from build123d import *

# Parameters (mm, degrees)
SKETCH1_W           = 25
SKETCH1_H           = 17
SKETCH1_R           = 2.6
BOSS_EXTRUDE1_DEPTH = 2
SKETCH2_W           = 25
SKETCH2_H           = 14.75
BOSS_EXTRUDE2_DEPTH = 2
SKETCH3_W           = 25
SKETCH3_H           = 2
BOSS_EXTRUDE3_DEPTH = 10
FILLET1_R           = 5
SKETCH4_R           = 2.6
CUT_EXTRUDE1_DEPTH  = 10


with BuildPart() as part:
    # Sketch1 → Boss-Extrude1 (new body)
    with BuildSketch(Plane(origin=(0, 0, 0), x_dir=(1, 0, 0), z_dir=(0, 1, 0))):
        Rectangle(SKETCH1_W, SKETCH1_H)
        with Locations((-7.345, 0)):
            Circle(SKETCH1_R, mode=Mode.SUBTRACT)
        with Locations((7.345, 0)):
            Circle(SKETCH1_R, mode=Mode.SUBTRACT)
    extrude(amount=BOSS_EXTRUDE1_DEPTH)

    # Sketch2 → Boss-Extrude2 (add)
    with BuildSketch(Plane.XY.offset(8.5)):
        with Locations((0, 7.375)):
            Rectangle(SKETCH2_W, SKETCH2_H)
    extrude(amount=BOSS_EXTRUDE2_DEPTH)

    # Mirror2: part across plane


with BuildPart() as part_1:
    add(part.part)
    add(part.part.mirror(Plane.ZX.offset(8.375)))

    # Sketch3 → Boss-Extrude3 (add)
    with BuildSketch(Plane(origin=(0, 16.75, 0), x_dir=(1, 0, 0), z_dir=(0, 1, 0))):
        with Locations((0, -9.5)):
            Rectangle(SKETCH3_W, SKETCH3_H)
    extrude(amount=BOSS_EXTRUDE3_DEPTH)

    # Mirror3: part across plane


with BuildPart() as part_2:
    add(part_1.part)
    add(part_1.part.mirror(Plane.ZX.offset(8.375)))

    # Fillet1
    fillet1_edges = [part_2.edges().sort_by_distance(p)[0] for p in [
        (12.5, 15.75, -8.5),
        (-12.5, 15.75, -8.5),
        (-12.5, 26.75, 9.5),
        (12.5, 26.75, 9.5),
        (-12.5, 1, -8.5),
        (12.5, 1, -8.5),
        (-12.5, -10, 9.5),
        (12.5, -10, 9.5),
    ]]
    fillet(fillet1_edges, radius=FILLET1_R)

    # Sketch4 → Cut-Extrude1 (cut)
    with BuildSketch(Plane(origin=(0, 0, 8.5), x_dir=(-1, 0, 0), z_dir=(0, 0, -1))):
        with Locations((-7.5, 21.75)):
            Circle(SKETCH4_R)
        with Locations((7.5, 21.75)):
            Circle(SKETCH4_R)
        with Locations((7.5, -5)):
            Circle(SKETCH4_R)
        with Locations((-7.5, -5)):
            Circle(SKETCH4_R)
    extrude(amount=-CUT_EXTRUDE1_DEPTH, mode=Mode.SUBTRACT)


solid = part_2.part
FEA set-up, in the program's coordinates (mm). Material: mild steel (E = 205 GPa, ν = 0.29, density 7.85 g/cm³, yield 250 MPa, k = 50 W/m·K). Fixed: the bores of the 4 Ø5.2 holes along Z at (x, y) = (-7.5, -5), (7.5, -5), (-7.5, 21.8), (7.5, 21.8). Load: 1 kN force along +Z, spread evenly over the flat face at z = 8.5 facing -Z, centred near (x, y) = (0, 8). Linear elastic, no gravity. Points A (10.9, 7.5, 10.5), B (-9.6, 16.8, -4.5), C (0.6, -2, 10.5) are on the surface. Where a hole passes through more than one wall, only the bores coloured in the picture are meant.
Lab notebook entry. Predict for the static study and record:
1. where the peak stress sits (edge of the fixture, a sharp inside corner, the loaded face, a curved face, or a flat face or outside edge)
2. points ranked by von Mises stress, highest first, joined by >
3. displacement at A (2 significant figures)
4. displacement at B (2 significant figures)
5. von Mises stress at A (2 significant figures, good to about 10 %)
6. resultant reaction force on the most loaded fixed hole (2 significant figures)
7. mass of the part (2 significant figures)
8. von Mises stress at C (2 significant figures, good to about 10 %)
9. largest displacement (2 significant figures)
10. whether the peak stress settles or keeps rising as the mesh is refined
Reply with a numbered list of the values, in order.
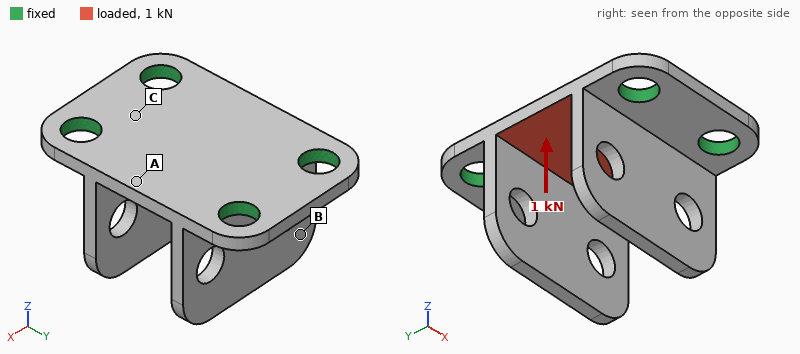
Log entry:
1. edge of the fixture
2. A > C > B
3. 16 µm
4. 27 µm
5. 93 MPa
6. 250 N
7. 24 g
8. 55 MPa
9. 35 µm
10. keeps rising
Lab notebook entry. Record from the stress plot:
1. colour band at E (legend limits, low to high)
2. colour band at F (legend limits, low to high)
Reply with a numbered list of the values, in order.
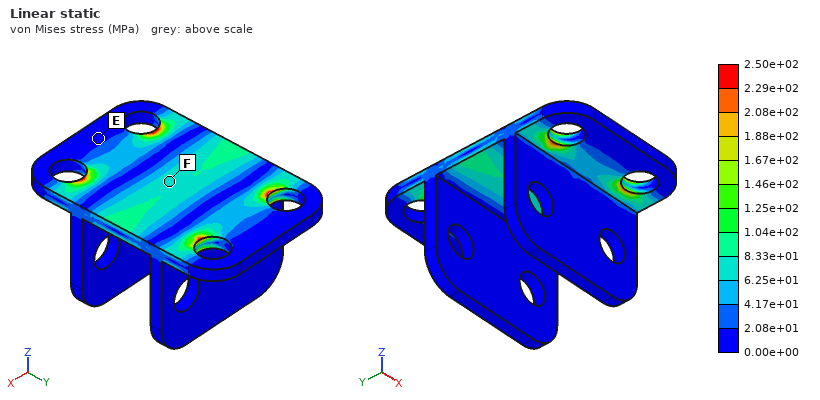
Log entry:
1. 0.00e+00 to 2.08e+01 MPa
2. 6.25e+01 to 8.33e+01 MPa
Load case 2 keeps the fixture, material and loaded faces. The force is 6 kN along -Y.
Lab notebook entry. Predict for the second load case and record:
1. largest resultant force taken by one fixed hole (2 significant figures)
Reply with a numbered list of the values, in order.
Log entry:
1. 1.5 kN
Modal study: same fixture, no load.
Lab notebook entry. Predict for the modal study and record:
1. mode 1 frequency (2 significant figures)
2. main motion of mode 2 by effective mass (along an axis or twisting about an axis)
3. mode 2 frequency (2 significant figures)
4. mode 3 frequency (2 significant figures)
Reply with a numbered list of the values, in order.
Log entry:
1. 4400 Hz
2. along Y
3. 5100 Hz
4. 9300 Hz
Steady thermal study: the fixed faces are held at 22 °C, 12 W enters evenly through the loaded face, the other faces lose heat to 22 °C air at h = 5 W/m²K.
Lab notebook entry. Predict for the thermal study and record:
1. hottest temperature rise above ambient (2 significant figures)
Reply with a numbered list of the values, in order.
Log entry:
1. 21 K
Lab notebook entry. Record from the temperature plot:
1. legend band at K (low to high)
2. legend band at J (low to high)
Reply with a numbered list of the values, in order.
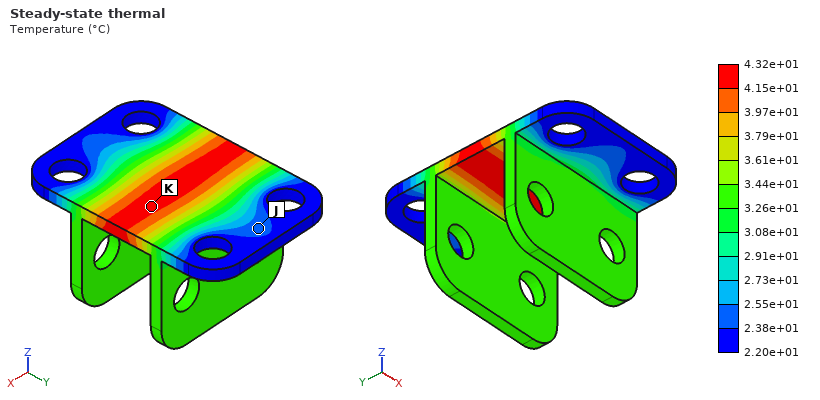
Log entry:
1. 4.15e+01 to 4.32e+01 °C
2. 2.38e+01 to 2.55e+01 °C
